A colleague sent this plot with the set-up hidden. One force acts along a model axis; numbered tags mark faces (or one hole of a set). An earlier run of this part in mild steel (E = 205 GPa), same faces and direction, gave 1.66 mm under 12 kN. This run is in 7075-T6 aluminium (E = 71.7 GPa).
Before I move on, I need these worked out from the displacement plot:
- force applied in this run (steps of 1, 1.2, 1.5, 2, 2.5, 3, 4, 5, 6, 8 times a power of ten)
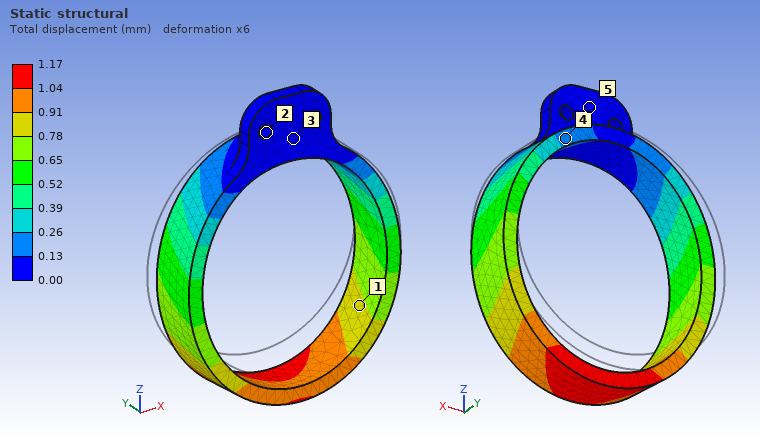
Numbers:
3 kN
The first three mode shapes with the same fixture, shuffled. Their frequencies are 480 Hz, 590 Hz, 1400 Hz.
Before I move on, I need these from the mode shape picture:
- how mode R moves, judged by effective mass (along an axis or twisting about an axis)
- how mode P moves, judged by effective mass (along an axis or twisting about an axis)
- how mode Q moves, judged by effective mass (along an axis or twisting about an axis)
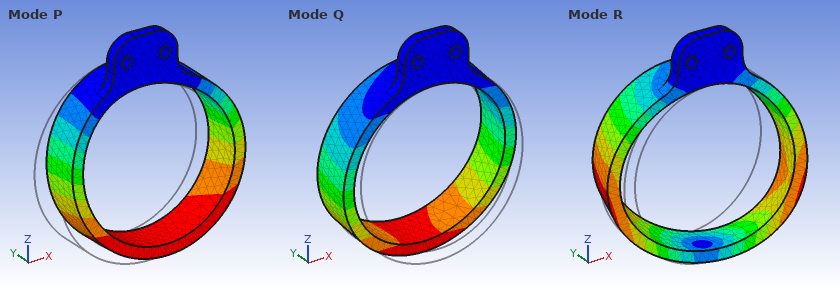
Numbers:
twisting about Z
along X
along Y
